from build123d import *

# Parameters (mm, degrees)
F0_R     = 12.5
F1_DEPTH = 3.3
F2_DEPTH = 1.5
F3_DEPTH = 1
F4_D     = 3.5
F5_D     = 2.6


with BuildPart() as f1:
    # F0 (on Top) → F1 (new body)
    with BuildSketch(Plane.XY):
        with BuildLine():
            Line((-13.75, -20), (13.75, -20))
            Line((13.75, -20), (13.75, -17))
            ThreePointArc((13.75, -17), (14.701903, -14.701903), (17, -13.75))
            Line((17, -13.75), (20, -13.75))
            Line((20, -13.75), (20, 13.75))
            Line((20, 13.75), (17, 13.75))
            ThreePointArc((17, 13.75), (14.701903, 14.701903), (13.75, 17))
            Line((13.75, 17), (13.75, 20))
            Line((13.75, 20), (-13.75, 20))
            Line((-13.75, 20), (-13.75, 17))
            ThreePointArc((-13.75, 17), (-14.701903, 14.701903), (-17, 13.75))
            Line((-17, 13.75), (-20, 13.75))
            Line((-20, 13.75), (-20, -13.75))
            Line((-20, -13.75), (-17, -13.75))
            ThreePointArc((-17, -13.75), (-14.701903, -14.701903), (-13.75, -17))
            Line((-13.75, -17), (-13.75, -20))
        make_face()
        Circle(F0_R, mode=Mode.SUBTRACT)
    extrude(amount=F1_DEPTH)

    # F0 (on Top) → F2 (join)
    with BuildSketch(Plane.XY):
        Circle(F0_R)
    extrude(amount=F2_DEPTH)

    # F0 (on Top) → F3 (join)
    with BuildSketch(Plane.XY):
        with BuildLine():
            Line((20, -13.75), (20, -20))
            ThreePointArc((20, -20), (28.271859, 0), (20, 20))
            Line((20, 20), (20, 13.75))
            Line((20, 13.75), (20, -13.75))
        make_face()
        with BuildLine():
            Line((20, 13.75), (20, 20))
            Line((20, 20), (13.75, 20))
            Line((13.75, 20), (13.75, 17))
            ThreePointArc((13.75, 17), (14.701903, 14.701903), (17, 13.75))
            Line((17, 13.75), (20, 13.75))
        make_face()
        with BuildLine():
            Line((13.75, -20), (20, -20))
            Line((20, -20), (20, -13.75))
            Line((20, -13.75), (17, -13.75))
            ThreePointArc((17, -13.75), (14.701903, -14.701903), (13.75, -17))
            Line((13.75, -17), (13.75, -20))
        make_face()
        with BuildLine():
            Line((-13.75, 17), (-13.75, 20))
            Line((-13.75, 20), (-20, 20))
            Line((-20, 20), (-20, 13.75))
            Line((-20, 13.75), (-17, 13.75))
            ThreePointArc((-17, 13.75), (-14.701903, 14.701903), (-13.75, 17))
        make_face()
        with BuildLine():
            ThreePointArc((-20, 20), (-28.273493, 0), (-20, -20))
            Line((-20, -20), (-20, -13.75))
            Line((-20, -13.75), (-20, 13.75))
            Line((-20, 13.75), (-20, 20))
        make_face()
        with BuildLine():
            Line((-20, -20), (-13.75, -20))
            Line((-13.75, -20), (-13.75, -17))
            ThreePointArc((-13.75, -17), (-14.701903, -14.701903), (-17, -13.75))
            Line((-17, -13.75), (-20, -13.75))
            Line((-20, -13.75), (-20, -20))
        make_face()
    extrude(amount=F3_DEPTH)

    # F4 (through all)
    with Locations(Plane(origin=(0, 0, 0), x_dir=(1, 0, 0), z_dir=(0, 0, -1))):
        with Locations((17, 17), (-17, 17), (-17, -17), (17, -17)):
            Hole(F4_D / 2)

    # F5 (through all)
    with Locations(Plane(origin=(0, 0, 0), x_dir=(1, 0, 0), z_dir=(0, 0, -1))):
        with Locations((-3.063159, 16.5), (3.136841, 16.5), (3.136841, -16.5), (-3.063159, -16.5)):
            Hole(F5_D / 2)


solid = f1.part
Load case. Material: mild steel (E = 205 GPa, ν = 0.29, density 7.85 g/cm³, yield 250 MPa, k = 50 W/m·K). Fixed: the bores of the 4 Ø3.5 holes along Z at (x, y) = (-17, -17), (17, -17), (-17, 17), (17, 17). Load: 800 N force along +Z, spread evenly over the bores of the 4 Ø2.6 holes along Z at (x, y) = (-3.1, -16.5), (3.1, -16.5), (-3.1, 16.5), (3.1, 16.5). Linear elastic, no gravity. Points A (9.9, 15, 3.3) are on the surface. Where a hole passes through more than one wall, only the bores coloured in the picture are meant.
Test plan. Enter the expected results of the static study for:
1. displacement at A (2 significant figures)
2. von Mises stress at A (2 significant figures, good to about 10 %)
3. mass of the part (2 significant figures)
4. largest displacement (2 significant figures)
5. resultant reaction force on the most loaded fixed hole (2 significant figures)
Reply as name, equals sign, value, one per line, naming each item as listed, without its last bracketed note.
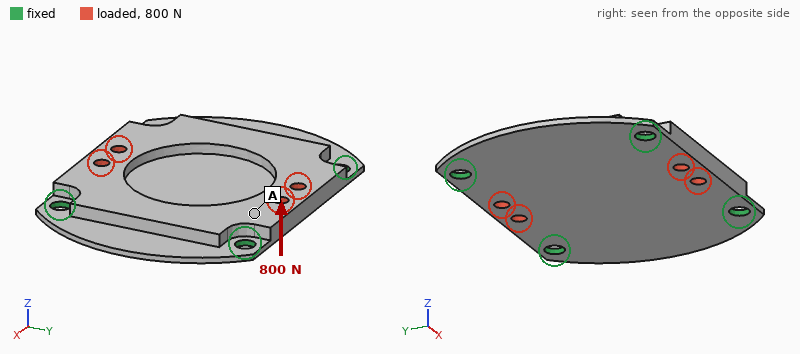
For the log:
displacement at A = 13 µm
von Mises stress at A = 35 MPa
mass of the part = 35 g
largest displacement = 27 µm
resultant reaction force on the most loaded fixed hole = 490 N
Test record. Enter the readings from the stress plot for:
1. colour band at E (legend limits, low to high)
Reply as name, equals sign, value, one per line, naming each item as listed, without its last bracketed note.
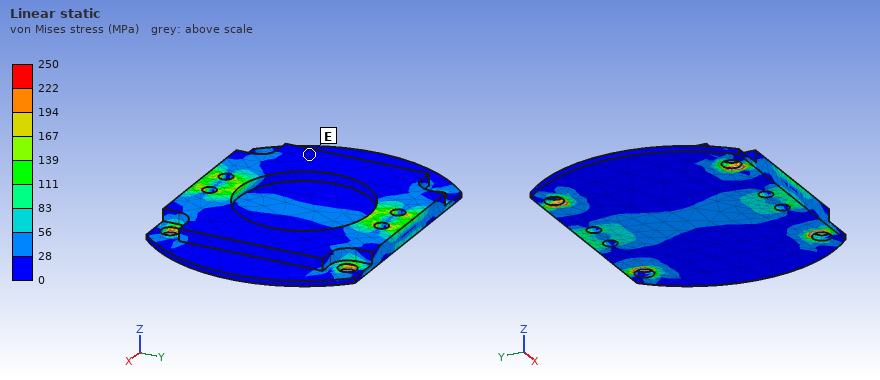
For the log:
colour band at E = 0 to 28 MPa
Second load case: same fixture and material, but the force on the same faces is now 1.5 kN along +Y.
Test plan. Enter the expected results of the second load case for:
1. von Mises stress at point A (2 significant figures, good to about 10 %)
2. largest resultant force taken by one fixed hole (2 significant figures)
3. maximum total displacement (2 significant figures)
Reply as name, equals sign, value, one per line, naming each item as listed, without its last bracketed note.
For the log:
von Mises stress at point A = 13 MPa
largest resultant force taken by one fixed hole = 390 N
maximum total displacement = 3.7 µm
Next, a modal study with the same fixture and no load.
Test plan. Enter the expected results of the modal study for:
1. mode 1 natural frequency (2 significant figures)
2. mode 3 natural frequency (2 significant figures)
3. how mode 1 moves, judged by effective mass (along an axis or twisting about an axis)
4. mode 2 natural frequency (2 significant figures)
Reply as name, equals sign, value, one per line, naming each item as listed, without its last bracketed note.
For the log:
mode 1 natural frequency = 7100 Hz
mode 3 natural frequency = 9200 Hz
how mode 1 moves, judged by effective mass = along Z
mode 2 natural frequency = 8900 Hz
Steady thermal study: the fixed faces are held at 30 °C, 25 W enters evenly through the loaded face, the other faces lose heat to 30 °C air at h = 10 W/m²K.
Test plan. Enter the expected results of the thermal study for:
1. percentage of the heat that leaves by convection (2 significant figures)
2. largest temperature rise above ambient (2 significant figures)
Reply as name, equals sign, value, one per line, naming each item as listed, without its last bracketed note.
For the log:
percentage of the heat that leaves by convection = 6.3 %
largest temperature rise above ambient = 72 K
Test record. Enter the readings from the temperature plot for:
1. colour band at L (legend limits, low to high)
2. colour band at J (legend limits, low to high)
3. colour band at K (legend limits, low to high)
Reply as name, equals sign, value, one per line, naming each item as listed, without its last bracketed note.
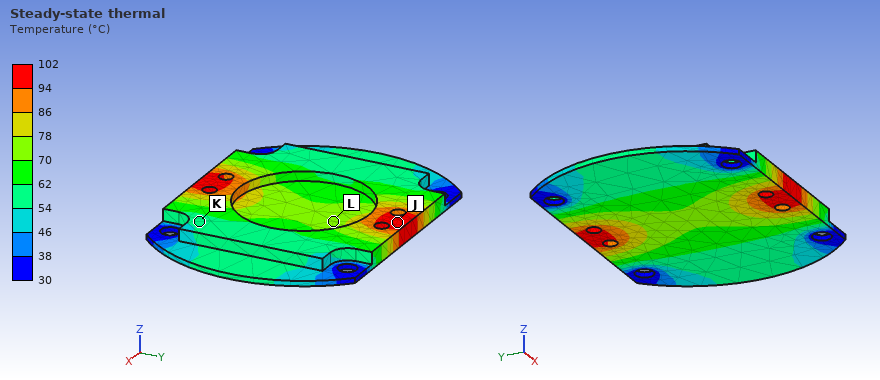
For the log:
colour band at L = 70 to 78 °C
colour band at J = 94 to 102 °C
colour band at K = 54 to 62 °C
